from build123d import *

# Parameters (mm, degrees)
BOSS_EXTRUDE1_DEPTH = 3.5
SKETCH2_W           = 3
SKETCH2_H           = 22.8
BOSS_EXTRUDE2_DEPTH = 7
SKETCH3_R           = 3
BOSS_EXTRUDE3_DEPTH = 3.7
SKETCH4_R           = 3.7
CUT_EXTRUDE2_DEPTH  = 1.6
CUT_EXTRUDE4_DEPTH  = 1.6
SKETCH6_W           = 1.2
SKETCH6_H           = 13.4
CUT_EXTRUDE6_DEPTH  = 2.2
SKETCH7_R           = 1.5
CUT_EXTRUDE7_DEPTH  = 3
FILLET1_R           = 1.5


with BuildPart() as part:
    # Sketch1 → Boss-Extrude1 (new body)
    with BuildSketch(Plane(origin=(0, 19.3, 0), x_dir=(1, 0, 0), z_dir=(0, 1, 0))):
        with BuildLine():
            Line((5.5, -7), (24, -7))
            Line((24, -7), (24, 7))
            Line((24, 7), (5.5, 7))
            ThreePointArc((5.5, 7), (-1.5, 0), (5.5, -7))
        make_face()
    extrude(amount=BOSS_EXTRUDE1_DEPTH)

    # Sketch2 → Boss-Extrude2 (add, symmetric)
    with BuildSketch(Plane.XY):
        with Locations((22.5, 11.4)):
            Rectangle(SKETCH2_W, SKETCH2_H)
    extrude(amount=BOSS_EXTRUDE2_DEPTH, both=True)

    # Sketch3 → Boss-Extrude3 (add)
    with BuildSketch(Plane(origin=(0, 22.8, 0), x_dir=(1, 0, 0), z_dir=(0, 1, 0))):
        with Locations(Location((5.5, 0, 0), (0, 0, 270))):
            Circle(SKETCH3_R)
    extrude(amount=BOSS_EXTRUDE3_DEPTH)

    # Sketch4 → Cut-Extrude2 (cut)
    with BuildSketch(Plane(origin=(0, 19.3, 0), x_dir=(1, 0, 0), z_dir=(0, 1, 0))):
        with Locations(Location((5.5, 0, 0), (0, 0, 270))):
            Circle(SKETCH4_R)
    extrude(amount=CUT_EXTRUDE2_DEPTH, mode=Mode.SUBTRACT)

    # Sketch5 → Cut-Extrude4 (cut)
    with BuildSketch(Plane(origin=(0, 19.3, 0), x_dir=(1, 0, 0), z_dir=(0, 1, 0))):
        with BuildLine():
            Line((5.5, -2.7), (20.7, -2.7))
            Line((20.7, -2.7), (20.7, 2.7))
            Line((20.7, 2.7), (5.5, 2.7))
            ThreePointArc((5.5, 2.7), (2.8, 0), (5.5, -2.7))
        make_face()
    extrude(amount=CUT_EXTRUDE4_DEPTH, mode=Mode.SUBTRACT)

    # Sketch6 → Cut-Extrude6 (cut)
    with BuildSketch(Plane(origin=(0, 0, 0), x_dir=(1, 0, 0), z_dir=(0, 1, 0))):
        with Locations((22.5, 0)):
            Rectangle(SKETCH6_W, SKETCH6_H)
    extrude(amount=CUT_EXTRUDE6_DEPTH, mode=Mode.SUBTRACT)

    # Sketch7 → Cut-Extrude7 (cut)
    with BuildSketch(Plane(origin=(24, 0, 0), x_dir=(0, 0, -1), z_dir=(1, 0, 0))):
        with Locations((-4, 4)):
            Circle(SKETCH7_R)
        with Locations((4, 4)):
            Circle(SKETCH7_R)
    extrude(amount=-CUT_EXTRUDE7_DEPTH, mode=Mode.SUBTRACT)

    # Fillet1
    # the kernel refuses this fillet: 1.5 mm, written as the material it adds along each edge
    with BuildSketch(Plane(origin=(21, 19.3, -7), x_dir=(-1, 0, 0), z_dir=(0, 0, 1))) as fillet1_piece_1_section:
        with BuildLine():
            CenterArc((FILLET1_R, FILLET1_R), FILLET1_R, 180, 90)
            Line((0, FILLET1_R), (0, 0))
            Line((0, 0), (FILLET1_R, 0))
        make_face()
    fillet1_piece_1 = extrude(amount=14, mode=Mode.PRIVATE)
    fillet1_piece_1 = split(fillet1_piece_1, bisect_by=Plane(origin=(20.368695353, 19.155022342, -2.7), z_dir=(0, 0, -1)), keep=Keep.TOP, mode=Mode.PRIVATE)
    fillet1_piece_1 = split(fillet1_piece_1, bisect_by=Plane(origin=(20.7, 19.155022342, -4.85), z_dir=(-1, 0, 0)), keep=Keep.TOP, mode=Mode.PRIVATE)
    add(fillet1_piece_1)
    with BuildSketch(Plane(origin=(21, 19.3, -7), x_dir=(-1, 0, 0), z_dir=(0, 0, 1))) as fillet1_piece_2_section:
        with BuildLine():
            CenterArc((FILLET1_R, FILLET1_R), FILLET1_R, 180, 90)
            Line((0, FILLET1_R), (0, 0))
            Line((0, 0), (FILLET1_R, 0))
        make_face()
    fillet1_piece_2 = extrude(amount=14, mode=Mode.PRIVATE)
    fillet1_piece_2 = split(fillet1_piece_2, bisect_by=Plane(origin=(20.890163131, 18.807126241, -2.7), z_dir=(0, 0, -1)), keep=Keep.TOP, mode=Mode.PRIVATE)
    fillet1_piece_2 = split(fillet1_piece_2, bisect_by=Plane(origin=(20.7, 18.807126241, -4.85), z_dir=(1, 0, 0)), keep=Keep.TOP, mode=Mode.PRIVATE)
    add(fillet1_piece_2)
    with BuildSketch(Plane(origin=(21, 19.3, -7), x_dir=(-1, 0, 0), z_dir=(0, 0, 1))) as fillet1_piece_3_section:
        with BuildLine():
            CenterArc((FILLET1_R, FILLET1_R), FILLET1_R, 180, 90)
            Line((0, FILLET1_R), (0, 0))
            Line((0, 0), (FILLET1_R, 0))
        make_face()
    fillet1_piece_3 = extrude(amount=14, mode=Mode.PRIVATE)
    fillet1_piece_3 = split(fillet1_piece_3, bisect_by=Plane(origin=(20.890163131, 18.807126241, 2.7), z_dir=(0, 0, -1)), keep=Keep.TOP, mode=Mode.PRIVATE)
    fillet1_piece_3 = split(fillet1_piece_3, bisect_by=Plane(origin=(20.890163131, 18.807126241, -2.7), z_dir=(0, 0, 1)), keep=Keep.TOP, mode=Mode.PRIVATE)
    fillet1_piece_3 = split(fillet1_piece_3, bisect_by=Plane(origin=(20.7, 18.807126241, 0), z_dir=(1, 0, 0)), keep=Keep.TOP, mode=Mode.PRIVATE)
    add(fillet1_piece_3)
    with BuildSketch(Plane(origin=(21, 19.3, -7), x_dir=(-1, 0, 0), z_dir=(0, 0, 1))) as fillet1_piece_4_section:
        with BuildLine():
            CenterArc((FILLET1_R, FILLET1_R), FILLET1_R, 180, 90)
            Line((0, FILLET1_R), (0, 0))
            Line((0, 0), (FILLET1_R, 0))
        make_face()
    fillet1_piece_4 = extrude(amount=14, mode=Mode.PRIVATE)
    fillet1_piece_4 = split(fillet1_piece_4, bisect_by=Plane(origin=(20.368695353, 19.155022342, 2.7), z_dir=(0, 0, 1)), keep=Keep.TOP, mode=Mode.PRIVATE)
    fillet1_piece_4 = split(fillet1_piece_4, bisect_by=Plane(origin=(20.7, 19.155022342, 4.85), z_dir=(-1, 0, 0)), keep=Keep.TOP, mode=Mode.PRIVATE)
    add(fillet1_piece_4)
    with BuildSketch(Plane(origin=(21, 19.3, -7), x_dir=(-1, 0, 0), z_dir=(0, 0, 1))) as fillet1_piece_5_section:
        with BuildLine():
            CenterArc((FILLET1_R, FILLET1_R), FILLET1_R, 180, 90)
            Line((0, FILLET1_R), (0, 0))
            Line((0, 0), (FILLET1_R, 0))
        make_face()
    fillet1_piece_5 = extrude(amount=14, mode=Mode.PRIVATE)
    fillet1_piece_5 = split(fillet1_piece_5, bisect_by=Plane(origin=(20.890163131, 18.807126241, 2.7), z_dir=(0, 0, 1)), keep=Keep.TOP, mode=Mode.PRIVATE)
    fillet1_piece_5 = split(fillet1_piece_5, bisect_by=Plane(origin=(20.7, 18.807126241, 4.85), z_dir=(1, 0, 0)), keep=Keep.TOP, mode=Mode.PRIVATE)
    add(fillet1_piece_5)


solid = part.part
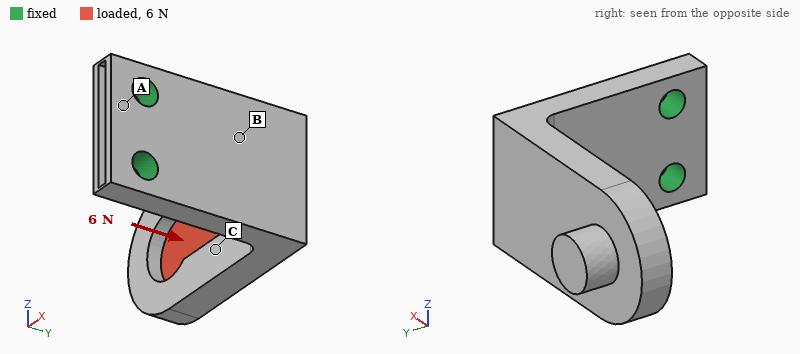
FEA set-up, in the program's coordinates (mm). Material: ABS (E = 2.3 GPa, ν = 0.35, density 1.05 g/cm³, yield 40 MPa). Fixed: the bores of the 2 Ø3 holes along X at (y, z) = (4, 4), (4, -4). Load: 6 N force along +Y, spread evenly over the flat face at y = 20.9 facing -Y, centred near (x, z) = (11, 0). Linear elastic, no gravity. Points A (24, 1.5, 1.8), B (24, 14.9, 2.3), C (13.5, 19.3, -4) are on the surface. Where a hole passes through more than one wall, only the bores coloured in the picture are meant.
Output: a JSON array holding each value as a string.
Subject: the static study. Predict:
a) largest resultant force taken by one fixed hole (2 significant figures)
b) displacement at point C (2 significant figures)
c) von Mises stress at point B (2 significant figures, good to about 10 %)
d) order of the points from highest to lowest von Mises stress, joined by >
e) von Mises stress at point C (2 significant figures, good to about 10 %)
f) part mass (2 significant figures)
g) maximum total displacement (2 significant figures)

["3.0 N", "0.17 mm", "2.9 MPa", "B > C > A", "1.1 MPa", "1.9 g", "0.45 mm"]
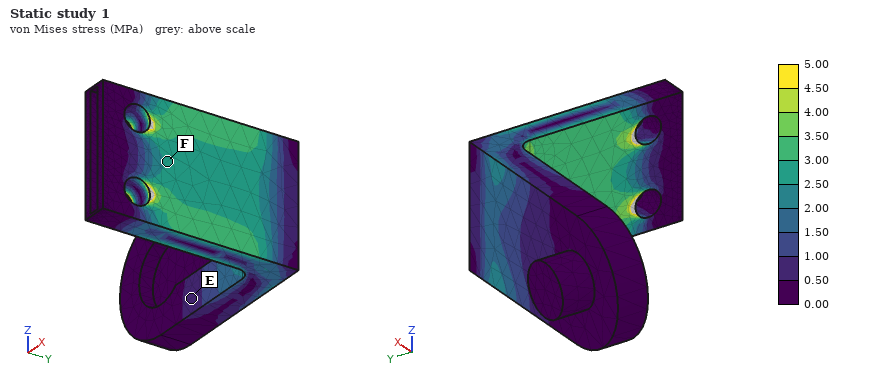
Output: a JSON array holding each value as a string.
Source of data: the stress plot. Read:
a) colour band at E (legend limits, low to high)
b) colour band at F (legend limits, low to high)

["0.50 to 1.00 MPa", "2.50 to 3.00 MPa"]
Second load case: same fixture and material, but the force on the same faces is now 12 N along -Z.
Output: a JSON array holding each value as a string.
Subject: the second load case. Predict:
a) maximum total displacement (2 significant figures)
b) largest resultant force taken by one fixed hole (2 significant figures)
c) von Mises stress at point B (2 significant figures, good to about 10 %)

["0.41 mm", "25 N", "4.4 MPa"]
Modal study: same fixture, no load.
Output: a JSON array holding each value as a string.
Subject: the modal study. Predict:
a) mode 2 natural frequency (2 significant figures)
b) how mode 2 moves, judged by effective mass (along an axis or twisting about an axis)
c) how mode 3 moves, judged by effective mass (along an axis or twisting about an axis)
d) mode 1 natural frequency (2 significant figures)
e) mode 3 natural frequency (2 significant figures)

["970 Hz", "along Z", "along X", "590 Hz", "1900 Hz"]
